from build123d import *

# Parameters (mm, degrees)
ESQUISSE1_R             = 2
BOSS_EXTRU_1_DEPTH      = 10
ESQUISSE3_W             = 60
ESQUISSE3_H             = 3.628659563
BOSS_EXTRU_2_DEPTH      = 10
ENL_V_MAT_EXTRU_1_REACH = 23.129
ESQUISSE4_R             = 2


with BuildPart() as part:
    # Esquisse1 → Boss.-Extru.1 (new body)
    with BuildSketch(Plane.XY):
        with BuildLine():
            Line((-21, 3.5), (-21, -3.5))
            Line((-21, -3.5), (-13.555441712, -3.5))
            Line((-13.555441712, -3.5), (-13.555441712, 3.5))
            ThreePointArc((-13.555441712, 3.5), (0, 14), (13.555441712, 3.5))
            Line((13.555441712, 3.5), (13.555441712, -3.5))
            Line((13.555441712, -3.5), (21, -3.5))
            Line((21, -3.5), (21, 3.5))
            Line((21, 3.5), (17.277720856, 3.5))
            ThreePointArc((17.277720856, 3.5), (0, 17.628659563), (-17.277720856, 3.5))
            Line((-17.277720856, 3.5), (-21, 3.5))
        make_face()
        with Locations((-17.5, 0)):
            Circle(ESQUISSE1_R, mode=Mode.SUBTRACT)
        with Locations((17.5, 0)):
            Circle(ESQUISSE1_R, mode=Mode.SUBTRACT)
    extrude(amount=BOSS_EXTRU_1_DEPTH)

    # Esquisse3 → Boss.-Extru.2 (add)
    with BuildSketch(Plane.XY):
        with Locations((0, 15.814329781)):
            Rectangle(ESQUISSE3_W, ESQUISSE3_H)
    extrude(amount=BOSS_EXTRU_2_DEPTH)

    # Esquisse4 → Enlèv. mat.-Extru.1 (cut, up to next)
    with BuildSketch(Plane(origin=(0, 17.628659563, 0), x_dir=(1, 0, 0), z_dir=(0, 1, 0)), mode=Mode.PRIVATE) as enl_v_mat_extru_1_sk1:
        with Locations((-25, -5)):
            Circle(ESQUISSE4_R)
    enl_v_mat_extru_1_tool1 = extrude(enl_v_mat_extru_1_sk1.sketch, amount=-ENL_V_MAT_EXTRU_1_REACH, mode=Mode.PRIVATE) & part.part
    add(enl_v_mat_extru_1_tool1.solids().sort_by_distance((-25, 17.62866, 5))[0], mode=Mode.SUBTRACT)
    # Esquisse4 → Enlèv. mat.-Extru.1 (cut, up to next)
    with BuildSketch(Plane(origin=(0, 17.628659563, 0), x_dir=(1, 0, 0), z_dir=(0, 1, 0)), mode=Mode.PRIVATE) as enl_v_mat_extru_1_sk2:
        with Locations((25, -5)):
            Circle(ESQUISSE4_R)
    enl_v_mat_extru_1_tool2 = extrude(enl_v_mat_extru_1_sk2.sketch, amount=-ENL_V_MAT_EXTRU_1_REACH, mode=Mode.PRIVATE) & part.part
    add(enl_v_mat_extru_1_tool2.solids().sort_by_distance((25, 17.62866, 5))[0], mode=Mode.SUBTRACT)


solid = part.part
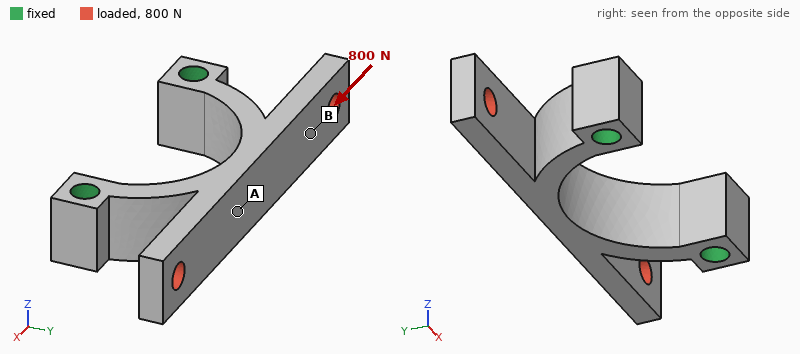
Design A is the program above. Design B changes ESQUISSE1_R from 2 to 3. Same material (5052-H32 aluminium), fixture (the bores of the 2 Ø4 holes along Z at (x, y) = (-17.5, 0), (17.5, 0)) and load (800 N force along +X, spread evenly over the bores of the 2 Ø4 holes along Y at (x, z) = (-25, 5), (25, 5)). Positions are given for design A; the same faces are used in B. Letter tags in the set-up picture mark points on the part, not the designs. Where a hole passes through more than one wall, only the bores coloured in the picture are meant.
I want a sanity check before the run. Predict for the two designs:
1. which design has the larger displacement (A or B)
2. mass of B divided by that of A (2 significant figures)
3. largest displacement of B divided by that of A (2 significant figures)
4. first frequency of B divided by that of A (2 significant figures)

A
0.92
0.90
1.0
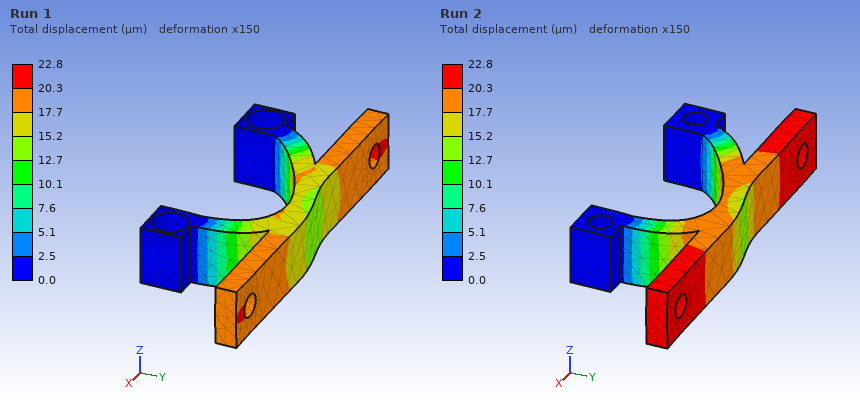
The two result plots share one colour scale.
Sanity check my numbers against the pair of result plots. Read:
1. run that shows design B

Run 1
